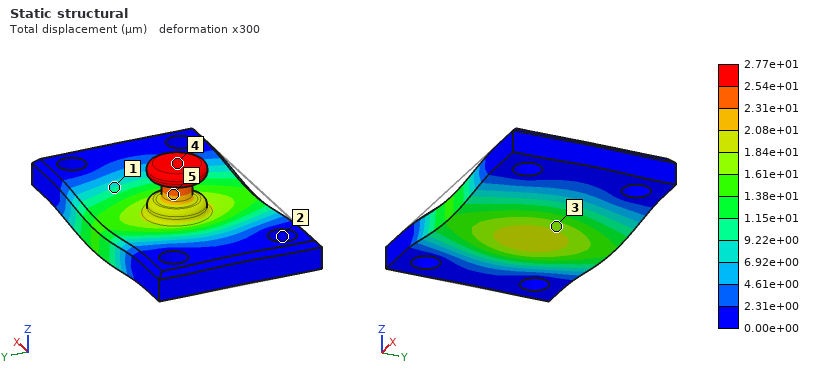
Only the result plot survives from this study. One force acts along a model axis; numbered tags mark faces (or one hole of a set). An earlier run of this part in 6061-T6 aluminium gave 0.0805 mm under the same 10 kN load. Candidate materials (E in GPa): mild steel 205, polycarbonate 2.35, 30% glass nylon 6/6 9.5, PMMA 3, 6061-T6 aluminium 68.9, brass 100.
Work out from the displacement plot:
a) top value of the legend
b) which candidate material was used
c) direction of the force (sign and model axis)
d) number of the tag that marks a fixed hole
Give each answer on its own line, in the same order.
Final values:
2.77e+01 µm
mild steel
-Z
2
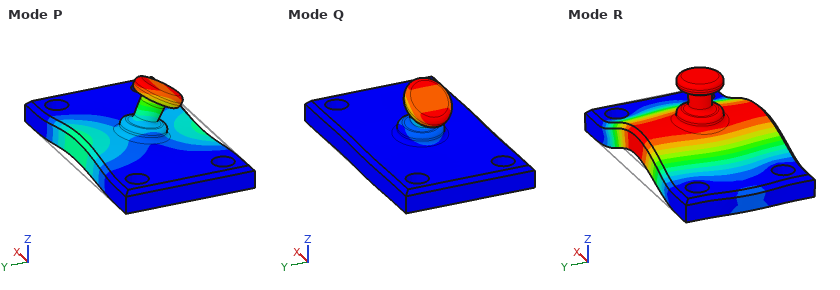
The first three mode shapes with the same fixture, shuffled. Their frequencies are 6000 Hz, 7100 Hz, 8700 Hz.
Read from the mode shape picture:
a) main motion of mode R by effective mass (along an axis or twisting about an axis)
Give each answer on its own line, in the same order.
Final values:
along Z
